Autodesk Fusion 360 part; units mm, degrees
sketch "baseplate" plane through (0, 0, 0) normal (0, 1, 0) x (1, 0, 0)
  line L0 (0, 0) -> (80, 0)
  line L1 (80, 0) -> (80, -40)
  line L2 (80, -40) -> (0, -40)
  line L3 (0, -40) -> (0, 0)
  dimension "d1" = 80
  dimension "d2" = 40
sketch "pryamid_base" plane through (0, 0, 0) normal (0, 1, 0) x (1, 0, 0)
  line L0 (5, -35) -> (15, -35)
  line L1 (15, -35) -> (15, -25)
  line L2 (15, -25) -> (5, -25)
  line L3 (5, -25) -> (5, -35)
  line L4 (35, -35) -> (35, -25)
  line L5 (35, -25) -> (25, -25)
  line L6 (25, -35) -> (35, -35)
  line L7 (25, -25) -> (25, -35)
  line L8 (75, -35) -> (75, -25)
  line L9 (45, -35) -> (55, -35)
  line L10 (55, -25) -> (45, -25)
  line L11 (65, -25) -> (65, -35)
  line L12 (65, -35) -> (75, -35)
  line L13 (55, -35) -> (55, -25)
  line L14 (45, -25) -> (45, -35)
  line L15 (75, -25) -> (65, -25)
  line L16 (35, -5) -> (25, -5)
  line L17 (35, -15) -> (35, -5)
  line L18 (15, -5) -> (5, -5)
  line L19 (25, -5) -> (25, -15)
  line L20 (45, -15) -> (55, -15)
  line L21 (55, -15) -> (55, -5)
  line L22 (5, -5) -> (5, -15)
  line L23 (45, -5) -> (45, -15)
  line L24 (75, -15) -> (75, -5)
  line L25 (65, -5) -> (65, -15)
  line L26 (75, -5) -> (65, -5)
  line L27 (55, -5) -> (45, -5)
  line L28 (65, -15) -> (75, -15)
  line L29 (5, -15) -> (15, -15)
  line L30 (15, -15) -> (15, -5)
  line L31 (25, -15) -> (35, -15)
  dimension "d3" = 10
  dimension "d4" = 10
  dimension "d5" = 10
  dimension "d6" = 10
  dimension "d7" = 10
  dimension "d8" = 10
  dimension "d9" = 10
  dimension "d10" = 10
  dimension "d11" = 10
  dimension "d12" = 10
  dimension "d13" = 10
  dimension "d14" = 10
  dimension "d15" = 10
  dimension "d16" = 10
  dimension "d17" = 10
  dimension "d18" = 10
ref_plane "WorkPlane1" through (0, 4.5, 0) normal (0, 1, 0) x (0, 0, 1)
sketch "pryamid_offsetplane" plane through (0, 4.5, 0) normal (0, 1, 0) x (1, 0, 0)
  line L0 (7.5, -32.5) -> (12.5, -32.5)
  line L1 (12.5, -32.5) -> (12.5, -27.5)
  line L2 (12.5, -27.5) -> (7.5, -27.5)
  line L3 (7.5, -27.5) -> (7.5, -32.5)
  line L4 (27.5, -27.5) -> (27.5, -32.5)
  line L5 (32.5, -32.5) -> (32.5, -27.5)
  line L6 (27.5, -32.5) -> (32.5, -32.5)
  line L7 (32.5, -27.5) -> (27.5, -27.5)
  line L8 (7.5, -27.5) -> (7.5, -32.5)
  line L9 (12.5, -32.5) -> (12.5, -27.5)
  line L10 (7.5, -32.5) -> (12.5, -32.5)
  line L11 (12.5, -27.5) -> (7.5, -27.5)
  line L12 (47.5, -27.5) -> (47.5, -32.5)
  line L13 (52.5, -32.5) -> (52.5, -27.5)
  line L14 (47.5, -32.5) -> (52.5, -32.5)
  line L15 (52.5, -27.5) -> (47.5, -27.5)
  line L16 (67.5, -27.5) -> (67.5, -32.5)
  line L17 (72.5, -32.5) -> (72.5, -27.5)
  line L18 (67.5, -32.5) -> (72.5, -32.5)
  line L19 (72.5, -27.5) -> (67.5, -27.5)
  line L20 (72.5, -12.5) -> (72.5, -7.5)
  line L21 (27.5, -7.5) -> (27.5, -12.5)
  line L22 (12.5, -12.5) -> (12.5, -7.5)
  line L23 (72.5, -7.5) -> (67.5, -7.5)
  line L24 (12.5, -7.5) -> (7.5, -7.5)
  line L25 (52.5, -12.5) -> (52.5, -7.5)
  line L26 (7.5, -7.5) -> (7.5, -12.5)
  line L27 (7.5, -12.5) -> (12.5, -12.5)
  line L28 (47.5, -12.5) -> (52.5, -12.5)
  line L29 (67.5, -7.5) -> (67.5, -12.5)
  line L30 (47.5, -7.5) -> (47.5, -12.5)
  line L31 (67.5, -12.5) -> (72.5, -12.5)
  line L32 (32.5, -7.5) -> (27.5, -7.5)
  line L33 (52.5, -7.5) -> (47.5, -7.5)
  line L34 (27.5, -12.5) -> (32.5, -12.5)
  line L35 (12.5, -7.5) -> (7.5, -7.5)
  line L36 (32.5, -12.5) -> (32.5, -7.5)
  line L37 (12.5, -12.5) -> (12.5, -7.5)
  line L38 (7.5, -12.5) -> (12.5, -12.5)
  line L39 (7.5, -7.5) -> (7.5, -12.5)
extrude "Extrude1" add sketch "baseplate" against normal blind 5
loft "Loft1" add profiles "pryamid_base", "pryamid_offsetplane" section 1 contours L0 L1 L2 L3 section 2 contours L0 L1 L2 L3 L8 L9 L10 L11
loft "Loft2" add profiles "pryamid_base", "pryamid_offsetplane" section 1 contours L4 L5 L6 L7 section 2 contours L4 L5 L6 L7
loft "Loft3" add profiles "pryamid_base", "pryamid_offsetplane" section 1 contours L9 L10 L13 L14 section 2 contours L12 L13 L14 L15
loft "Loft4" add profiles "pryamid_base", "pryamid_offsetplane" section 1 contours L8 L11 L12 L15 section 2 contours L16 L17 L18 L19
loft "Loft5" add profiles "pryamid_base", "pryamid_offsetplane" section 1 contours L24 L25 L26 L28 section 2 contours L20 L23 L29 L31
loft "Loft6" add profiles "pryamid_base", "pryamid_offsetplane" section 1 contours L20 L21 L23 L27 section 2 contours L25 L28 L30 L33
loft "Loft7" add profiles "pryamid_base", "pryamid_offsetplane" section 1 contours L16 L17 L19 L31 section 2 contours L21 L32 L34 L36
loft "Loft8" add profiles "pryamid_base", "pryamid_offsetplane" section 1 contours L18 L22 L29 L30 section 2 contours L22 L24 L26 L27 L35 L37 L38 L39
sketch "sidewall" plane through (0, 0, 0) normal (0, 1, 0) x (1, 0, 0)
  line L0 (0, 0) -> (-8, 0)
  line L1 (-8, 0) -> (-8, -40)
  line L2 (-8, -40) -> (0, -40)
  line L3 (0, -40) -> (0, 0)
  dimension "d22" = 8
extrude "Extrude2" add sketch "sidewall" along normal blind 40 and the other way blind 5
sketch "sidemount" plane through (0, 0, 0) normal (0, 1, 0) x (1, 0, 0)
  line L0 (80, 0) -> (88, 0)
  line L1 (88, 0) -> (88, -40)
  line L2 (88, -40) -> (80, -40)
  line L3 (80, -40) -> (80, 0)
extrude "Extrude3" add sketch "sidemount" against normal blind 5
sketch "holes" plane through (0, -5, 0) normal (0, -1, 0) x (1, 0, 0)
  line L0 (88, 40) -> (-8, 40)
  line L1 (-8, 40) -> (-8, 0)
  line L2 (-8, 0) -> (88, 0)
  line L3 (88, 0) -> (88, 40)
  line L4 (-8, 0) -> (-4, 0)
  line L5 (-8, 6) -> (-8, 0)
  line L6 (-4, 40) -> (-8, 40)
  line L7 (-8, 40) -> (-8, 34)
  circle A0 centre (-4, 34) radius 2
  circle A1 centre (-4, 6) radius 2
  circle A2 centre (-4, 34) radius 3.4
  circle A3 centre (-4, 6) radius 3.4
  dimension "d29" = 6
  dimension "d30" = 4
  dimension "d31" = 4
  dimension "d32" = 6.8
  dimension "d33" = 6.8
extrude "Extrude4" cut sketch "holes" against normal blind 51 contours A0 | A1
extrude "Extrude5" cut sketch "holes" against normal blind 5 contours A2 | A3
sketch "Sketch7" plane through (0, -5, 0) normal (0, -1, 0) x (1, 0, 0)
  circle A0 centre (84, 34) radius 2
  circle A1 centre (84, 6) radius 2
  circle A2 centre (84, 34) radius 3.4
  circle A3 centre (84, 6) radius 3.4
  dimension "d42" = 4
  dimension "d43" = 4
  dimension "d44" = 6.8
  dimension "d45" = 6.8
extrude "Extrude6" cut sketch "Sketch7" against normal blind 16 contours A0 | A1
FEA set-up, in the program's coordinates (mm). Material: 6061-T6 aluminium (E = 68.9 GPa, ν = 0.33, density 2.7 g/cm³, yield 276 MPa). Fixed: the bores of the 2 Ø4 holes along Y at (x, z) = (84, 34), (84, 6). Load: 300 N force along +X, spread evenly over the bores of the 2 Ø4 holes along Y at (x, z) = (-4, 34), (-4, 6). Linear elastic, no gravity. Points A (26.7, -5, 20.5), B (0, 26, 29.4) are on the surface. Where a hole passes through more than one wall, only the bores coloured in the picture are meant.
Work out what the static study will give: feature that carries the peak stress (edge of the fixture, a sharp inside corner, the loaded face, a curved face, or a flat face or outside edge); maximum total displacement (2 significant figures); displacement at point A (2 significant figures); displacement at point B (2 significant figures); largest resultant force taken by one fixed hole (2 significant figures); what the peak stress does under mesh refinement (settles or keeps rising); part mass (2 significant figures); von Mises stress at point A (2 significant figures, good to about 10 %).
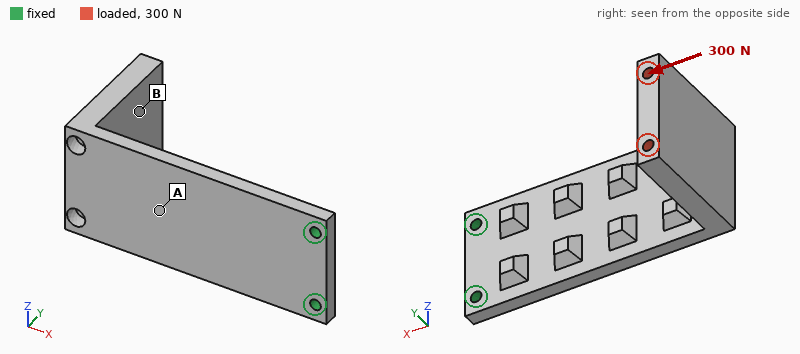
edge of the fixture
1.1 mm
0.35 mm
0.87 mm
150 N
keeps rising
88 g
29 MPa
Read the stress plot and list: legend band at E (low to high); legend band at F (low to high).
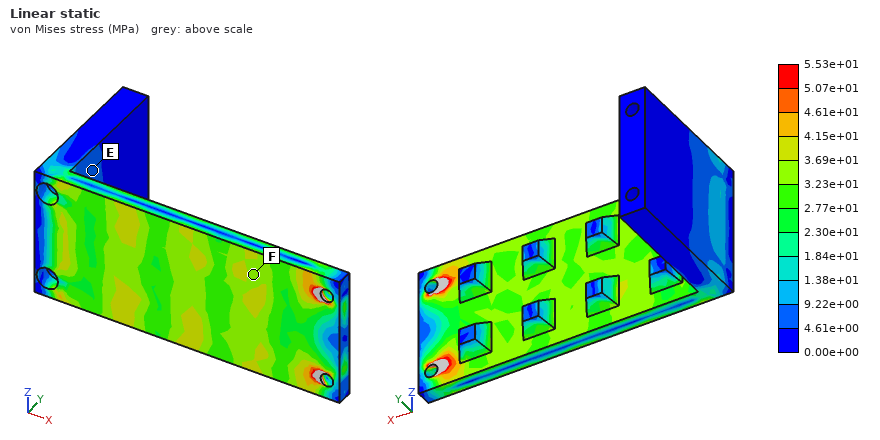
4.61e+00 to 9.22e+00 MPa
3.23e+01 to 3.69e+01 MPa
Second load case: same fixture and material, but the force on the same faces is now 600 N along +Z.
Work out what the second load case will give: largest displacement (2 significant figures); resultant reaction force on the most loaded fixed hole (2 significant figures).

0.93 mm
1.9 kN
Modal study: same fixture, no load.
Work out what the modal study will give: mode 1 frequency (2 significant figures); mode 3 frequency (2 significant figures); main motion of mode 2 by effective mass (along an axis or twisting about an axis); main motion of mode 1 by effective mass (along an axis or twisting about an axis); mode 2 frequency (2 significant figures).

260 Hz
1200 Hz
along Z
along Y
800 Hz
